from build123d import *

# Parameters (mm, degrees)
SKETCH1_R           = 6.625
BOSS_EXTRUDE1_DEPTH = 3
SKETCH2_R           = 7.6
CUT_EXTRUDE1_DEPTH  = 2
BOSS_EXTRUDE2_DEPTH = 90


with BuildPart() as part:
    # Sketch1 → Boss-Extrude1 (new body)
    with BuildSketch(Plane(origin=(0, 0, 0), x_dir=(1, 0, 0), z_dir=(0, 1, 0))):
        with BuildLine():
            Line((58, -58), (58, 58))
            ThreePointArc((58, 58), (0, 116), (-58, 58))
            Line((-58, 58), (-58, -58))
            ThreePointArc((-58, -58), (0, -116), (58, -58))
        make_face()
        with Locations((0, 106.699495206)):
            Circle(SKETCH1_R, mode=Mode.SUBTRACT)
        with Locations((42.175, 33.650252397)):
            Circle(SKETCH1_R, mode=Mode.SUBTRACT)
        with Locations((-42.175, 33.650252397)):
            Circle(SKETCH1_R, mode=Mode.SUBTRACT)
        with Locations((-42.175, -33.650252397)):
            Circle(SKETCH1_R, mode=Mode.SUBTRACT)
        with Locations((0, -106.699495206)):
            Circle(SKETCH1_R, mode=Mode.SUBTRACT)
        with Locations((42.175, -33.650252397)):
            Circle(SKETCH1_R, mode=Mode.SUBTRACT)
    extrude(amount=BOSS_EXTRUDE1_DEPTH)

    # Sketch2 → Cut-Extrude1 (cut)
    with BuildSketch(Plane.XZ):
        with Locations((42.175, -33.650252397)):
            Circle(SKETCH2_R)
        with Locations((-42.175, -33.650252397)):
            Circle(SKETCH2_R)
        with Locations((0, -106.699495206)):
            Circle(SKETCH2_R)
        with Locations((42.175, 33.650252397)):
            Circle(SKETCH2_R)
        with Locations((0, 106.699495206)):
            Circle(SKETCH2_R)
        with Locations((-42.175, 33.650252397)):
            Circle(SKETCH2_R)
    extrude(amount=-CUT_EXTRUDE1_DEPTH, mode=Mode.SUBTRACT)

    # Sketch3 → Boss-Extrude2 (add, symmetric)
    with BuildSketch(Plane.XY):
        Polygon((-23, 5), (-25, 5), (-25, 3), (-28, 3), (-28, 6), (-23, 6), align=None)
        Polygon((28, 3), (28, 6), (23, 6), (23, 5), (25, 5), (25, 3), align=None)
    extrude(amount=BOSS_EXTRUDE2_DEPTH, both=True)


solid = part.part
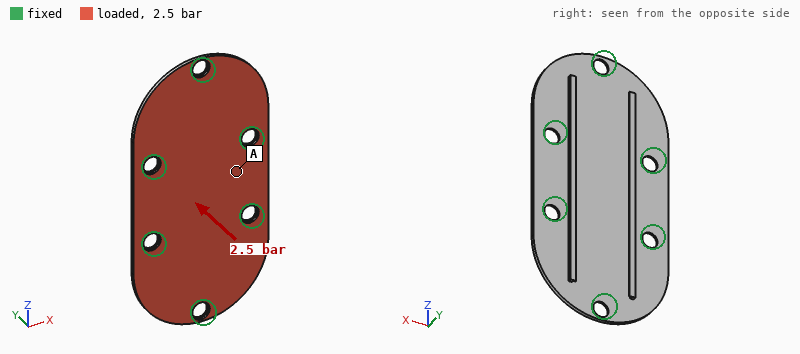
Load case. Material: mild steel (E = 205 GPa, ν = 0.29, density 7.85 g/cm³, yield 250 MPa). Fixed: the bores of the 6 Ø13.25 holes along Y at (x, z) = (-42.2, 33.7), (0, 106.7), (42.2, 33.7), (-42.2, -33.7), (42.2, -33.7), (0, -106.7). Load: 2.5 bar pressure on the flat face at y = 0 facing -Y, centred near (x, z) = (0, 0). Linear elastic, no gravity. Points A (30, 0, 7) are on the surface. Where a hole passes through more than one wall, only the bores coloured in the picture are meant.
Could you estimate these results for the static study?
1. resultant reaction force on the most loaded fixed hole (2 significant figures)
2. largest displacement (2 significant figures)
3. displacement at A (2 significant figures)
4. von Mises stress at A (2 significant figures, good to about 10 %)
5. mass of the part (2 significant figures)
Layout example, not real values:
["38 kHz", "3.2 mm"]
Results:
["1.5 kN", "0.13 mm", "0.033 mm", "32 MPa", "570 g"]
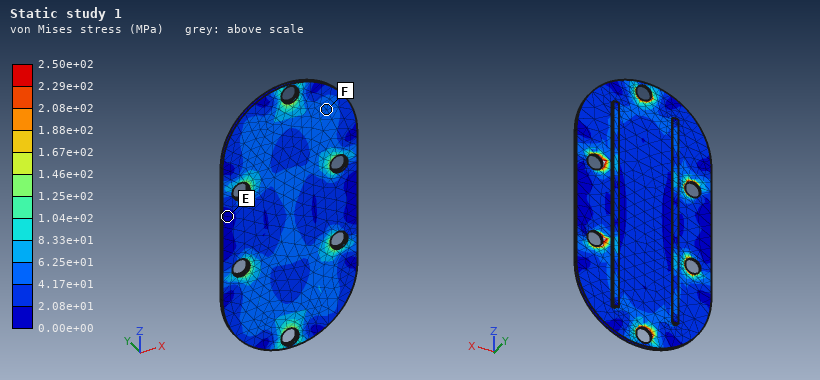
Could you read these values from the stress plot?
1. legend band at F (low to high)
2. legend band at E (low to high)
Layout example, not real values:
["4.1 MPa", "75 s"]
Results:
["4.17e+01 to 6.25e+01 MPa", "0.00e+00 to 2.08e+01 MPa"]
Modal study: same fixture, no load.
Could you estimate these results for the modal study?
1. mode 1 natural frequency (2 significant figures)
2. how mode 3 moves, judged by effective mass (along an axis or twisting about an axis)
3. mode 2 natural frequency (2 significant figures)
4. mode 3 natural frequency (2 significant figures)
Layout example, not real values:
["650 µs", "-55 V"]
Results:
["1700 Hz", "along Y", "1700 Hz", "1800 Hz"]
